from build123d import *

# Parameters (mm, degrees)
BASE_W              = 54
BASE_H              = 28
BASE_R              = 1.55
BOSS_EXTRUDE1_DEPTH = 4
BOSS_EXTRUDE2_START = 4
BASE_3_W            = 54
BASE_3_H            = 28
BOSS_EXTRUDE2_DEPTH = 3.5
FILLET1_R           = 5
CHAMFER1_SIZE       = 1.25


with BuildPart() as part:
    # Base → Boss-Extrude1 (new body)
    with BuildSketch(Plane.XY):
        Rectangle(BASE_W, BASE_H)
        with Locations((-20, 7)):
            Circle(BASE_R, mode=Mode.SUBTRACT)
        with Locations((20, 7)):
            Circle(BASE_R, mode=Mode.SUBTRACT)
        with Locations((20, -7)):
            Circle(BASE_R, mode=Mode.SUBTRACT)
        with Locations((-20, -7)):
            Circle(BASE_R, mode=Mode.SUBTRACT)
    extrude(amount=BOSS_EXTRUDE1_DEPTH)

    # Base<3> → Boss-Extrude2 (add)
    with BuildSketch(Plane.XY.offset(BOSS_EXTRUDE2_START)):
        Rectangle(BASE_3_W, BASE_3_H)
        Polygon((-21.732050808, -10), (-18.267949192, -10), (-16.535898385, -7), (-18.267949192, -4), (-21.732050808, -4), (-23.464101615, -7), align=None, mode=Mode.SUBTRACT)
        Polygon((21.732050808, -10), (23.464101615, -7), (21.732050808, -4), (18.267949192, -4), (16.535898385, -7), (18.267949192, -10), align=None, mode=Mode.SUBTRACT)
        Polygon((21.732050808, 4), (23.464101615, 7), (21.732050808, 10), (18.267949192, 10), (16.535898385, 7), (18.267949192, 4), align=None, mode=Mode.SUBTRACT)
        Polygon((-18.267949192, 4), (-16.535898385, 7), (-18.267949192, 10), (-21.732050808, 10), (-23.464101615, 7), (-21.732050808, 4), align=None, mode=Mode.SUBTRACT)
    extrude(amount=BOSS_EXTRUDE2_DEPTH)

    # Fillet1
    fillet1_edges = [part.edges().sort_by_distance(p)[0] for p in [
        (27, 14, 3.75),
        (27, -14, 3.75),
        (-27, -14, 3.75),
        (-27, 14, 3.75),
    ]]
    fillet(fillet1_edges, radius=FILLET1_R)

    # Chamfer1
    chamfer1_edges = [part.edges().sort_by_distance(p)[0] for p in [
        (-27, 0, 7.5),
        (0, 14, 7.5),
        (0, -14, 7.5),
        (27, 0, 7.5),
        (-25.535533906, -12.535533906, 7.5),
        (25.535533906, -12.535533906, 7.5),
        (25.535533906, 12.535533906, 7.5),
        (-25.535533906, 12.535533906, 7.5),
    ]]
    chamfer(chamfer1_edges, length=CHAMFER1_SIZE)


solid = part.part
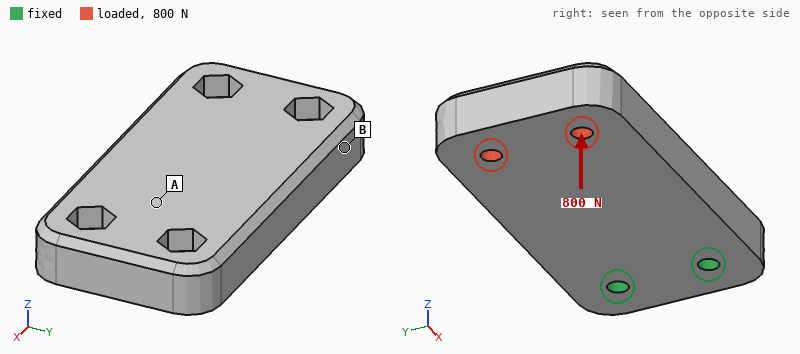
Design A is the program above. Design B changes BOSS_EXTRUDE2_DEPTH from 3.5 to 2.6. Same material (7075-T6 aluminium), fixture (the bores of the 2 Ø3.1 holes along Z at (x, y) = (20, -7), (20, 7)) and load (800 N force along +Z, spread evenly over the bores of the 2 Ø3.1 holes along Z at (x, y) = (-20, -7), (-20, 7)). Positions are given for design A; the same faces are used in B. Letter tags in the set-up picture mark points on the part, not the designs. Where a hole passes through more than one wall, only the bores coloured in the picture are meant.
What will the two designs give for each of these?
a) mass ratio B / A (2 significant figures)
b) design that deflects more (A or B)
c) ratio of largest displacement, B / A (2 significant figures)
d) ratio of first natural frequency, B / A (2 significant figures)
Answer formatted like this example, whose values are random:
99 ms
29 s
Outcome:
0.88
B
1.2
0.97
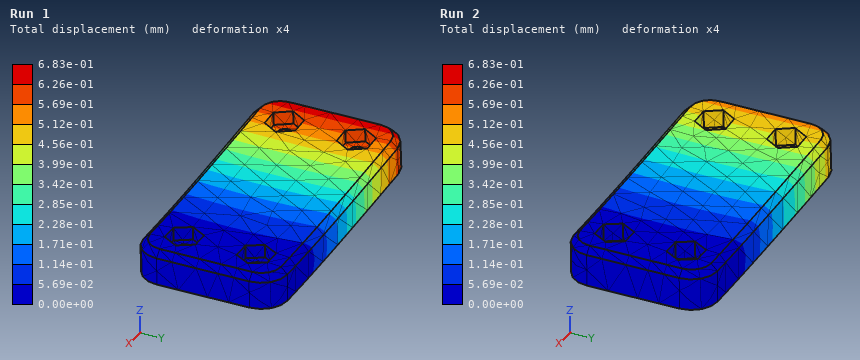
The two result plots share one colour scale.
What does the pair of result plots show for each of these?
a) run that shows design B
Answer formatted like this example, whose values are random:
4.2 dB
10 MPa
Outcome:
Run 1
